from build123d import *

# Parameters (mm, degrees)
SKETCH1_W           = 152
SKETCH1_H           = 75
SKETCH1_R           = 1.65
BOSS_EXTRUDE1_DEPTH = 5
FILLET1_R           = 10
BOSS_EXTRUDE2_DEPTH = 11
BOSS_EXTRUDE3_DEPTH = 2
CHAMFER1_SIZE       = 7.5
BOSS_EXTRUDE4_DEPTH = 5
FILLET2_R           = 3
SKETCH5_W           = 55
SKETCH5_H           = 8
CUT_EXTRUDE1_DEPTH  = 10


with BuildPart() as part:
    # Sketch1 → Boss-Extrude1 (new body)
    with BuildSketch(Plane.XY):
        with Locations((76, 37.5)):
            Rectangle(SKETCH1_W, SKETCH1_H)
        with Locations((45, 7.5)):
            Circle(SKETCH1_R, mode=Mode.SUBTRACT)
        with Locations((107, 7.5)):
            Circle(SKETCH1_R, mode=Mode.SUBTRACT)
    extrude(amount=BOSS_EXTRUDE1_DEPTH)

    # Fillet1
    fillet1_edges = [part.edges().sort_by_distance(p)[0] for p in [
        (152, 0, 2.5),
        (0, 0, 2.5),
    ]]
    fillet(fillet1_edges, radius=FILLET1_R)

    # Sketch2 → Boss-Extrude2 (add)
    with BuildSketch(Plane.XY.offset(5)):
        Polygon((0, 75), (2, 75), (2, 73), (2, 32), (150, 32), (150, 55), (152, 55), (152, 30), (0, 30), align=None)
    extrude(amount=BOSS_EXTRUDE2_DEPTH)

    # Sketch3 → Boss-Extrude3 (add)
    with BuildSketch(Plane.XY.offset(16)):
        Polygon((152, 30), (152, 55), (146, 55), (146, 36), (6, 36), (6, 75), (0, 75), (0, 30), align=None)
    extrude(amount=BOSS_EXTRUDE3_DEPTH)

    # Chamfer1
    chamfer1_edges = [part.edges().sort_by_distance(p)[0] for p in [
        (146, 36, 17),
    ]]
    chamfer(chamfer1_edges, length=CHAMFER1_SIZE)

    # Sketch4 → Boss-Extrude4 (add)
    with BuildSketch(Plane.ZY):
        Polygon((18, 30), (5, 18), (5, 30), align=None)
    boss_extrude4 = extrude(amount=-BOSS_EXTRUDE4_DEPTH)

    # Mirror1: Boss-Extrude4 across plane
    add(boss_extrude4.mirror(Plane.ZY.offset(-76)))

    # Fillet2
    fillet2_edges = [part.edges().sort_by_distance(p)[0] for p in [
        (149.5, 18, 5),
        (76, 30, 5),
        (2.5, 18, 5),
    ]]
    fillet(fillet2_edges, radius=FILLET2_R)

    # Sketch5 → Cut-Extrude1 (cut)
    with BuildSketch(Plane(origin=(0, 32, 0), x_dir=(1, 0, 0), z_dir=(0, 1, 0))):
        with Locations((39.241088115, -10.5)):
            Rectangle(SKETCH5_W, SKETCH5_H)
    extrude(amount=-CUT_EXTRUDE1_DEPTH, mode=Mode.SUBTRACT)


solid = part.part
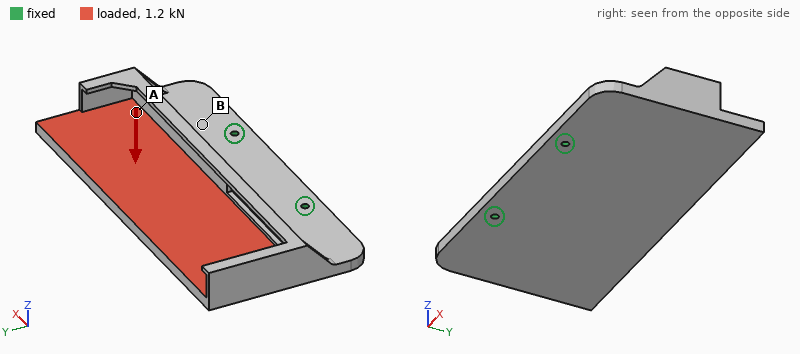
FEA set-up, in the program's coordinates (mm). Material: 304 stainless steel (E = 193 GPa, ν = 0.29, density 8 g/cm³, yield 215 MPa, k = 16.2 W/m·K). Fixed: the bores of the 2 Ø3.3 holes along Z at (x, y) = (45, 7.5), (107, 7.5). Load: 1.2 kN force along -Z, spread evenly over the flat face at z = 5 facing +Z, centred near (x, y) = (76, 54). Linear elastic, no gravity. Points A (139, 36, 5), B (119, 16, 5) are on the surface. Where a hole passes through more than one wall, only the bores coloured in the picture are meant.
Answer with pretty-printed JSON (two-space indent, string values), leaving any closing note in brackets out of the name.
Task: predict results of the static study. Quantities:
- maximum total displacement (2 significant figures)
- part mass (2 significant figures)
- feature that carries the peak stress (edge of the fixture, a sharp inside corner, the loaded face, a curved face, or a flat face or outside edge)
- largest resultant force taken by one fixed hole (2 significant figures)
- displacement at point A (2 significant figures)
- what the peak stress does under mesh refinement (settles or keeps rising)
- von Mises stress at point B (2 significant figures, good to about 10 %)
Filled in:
{
  "maximum total displacement": "0.42 mm",
  "part mass": "510 g",
  "feature that carries the peak stress": "edge of the fixture",
  "largest resultant force taken by one fixed hole": "620 N",
  "displacement at point A": "0.15 mm",
  "what the peak stress does under mesh refinement": "keeps rising",
  "von Mises stress at point B": "81 MPa"
}
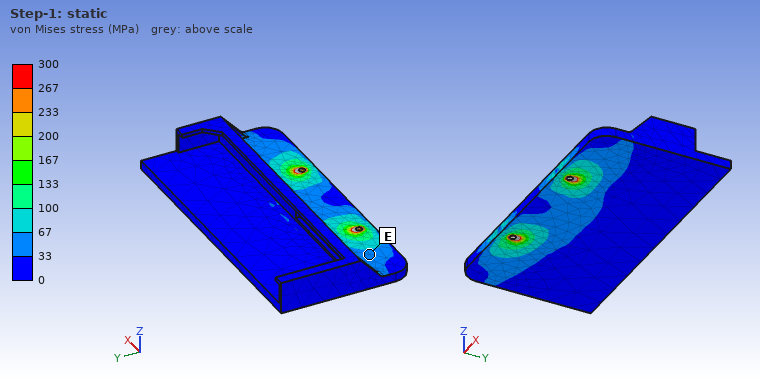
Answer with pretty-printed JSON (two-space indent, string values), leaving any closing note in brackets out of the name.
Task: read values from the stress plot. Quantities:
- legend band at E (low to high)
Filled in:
{
  "legend band at E": "33 to 67 MPa"
}
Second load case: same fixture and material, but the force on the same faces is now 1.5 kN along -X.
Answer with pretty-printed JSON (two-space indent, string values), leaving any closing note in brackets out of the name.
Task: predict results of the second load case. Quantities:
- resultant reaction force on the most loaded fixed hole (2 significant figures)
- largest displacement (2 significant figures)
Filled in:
{
  "resultant reaction force on the most loaded fixed hole": "1.3 kN",
  "largest displacement": "22 µm"
}
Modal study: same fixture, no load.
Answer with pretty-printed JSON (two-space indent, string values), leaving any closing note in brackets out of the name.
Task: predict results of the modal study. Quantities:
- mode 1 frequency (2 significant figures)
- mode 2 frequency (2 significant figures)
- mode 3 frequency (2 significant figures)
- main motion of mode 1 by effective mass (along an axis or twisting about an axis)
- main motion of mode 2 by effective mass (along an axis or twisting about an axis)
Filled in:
{
  "mode 1 frequency": "600 Hz",
  "mode 2 frequency": "810 Hz",
  "mode 3 frequency": "1800 Hz",
  "main motion of mode 1 by effective mass": "along Z",
  "main motion of mode 2 by effective mass": "twisting about Y"
}
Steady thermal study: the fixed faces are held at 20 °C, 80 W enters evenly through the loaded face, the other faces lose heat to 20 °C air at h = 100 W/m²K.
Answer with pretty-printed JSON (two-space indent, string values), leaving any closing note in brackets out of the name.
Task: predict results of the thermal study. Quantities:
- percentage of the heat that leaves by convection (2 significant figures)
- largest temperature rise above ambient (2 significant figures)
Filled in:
{
  "percentage of the heat that leaves by convection": "94 %",
  "largest temperature rise above ambient": "79 K"
}
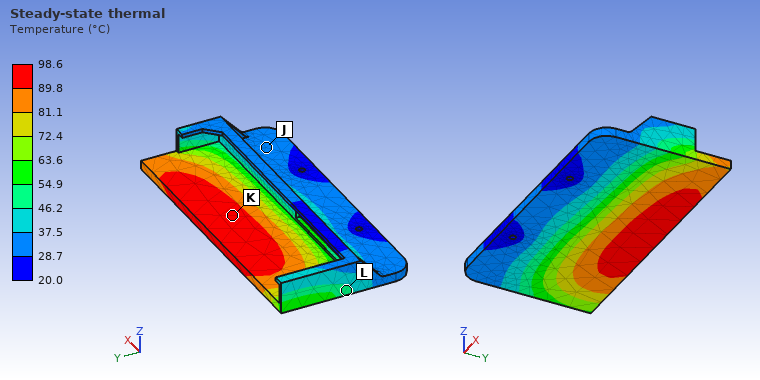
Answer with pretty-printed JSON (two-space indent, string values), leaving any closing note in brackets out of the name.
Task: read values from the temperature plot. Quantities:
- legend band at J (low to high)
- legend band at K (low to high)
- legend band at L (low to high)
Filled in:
{
  "legend band at J": "28.7 to 37.5 °C",
  "legend band at K": "89.8 to 98.6 °C",
  "legend band at L": "46.2 to 54.9 °C"
}
